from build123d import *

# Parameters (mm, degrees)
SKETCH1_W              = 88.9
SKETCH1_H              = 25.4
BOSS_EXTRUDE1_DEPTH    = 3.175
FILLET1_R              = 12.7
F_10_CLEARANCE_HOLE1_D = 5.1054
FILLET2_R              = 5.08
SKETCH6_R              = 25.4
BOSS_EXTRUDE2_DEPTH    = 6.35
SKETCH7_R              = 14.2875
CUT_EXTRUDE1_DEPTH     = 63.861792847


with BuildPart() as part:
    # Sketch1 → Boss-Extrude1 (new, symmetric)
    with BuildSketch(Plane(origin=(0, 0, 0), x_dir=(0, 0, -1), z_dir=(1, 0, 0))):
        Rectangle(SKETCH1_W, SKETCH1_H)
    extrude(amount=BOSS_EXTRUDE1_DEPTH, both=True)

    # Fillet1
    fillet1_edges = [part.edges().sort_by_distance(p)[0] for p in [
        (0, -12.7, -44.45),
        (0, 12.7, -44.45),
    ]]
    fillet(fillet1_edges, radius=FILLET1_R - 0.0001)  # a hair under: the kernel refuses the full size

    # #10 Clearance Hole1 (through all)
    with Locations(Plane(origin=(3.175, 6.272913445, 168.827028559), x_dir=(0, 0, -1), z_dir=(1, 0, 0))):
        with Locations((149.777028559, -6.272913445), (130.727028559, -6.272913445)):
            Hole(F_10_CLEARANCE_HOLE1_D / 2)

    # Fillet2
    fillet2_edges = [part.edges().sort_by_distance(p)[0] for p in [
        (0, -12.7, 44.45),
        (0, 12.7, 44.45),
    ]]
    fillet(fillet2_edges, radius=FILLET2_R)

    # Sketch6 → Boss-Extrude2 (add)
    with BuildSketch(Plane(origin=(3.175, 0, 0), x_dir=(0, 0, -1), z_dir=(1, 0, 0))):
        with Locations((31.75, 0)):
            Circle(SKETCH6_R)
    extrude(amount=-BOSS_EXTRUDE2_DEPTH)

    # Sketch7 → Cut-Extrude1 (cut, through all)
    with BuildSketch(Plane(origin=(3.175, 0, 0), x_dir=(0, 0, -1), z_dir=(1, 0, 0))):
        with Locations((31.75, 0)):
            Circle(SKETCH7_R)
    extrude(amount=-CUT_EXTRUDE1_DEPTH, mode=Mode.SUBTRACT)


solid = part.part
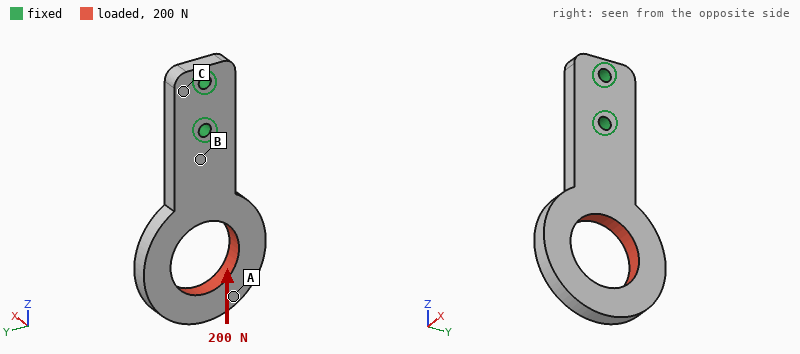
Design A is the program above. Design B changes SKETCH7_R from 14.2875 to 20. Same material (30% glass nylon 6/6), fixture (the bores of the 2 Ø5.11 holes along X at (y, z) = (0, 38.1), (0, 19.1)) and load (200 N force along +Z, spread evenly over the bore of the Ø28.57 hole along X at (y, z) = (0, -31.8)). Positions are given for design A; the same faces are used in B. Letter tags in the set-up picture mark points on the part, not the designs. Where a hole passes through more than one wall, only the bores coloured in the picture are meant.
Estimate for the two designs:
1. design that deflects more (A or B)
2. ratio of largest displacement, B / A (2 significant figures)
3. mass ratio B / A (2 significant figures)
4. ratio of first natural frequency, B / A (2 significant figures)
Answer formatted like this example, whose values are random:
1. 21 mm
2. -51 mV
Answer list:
1. B
2. 6.1
3. 0.77
4. 1.1
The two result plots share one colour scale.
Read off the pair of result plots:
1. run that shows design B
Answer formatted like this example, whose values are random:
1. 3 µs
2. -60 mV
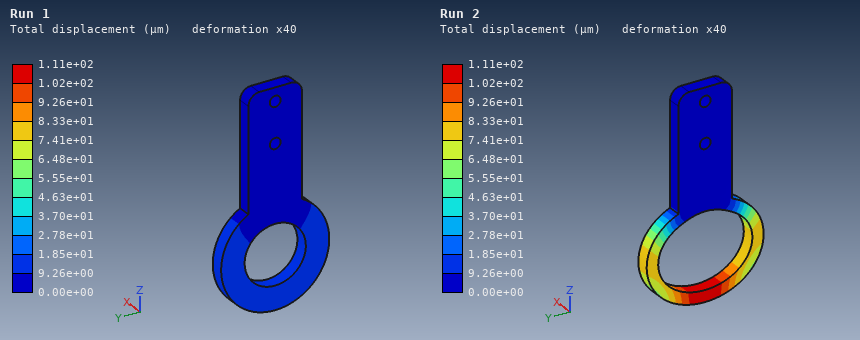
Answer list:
1. Run 2
